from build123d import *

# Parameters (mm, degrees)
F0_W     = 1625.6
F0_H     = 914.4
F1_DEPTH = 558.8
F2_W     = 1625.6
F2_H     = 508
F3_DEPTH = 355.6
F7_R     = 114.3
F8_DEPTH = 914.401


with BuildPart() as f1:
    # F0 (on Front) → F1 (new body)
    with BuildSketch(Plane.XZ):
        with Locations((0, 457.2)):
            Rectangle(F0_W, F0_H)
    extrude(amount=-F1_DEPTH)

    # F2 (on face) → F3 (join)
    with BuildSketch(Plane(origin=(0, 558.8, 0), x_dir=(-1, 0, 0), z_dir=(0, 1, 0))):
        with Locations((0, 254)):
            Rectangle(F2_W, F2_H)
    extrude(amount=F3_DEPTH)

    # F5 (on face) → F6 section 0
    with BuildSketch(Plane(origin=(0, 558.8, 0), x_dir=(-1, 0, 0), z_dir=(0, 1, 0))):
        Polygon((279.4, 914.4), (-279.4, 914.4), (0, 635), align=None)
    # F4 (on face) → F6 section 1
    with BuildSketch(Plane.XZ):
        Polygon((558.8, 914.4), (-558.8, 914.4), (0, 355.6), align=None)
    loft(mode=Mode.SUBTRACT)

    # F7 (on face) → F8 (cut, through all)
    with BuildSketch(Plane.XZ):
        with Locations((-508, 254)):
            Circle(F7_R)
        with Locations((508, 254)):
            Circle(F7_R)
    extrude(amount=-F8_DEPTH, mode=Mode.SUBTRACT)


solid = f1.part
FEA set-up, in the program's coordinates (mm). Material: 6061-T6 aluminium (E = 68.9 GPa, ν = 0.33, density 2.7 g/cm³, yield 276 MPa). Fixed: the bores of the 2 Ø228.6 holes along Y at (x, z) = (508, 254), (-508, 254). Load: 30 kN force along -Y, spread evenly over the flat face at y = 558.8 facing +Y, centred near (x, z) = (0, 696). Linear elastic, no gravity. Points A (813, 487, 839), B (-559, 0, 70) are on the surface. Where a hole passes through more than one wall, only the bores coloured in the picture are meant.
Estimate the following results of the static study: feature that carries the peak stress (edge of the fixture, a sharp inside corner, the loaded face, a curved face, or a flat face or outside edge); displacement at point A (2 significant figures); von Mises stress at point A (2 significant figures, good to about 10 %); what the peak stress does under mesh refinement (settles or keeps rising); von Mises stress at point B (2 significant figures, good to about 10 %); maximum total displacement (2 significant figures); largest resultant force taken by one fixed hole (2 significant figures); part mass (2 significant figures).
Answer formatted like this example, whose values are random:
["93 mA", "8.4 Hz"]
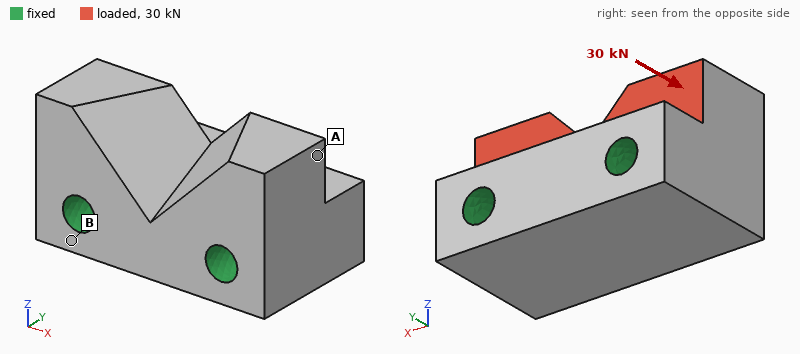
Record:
["edge of the fixture", "1.2 µm", "0.051 MPa", "keeps rising", "0.018 MPa", "1.7 µm", "15 kN", "2600 kg"]
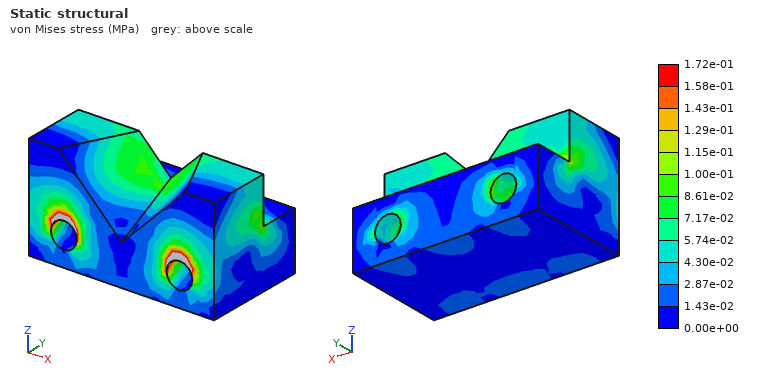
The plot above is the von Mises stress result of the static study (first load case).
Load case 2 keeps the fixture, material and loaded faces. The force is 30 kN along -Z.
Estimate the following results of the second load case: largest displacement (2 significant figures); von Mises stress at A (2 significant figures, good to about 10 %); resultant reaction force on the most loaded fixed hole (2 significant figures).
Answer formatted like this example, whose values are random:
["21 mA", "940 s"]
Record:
["1.6 µm", "0.041 MPa", "15 kN"]
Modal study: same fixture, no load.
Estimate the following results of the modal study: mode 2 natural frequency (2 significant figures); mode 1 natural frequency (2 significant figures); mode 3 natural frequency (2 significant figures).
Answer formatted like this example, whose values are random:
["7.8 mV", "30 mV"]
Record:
["1000 Hz", "930 Hz", "1000 Hz"]
